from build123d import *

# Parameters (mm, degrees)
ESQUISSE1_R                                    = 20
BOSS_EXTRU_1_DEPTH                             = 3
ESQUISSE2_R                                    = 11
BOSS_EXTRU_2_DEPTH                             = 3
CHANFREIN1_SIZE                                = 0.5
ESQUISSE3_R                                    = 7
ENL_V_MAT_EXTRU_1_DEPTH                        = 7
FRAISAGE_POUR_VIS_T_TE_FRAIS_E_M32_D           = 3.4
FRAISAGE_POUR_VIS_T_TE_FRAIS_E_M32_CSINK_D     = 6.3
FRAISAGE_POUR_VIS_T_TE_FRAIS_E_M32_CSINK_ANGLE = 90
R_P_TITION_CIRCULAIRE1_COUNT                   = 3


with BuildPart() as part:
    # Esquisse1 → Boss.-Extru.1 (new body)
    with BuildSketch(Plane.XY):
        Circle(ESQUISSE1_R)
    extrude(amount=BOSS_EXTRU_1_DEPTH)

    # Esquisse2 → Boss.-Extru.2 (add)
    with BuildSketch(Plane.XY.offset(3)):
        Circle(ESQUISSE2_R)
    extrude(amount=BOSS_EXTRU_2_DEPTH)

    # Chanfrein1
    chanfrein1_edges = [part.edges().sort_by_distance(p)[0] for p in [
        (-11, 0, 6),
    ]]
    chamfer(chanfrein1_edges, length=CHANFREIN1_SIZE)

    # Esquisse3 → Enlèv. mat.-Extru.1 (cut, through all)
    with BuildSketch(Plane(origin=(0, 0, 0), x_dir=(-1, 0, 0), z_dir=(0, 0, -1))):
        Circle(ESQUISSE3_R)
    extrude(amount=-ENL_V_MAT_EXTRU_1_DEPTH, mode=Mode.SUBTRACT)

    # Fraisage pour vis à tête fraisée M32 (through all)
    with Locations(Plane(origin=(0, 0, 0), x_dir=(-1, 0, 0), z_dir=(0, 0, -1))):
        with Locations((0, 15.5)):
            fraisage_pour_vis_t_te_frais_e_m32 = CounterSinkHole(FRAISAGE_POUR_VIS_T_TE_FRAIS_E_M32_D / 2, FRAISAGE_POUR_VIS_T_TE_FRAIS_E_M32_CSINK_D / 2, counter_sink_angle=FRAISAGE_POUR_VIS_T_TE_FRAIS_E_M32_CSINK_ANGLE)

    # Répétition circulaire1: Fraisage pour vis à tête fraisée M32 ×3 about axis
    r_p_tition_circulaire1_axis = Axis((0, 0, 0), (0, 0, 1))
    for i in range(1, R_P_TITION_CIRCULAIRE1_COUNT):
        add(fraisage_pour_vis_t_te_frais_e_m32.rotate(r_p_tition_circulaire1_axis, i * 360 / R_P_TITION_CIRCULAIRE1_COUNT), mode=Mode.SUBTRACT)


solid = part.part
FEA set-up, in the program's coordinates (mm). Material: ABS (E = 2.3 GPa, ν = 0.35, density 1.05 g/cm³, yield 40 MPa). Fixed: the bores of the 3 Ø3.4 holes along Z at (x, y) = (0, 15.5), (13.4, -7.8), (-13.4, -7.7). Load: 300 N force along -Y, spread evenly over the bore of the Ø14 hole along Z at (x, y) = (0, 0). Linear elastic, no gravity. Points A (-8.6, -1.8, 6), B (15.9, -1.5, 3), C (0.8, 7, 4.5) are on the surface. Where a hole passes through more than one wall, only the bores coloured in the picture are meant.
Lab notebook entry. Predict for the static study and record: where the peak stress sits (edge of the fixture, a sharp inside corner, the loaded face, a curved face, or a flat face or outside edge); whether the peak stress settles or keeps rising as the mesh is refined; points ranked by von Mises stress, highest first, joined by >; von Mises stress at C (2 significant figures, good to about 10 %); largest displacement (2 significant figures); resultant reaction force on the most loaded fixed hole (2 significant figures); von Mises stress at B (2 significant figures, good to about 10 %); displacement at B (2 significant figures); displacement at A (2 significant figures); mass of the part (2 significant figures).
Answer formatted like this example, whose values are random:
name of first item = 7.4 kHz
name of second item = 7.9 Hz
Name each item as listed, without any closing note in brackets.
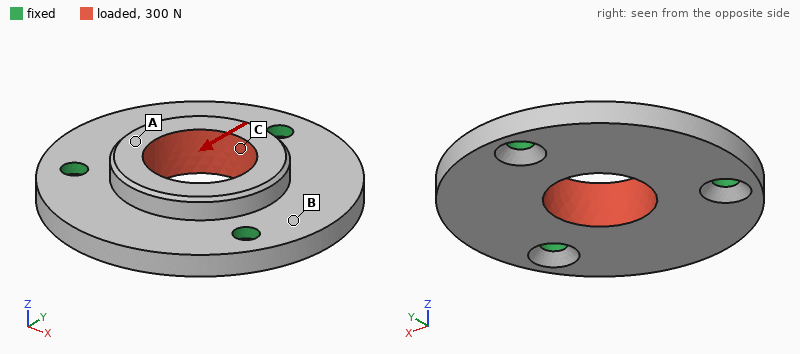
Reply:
where the peak stress sits = edge of the fixture
whether the peak stress settles or keeps rising as the mesh is refined = keeps rising
points ranked by von Mises stress, highest first, joined by > = C > B > A
von Mises stress at C = 3.5 MPa
largest displacement = 36 µm
resultant reaction force on the most loaded fixed hole = 100 N
von Mises stress at B = 2.3 MPa
displacement at B = 6.9 µm
displacement at A = 21 µm
mass of the part = 4.0 g
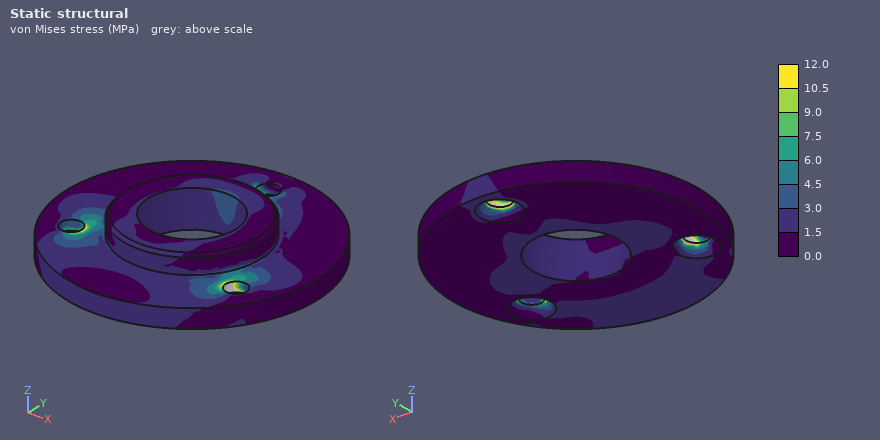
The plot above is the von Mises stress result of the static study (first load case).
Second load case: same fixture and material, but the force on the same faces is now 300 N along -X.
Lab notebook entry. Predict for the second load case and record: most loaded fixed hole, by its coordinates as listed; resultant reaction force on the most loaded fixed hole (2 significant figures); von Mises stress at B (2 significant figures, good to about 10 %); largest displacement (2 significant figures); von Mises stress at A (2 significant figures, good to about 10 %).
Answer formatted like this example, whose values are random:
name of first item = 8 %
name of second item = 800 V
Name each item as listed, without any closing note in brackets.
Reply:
most loaded fixed hole, by its coordinates as listed = (0, 15.5)
resultant reaction force on the most loaded fixed hole = 110 N
von Mises stress at B = 2.0 MPa
largest displacement = 32 µm
von Mises stress at A = 2.1 MPa
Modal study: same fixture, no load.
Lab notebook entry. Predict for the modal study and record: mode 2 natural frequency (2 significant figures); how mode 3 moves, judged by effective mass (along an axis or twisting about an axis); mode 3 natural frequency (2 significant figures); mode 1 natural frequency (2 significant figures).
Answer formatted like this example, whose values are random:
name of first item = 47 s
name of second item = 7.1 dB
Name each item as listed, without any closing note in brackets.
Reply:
mode 2 natural frequency = 3500 Hz
how mode 3 moves, judged by effective mass = along Z
mode 3 natural frequency = 4400 Hz
mode 1 natural frequency = 3500 Hz
